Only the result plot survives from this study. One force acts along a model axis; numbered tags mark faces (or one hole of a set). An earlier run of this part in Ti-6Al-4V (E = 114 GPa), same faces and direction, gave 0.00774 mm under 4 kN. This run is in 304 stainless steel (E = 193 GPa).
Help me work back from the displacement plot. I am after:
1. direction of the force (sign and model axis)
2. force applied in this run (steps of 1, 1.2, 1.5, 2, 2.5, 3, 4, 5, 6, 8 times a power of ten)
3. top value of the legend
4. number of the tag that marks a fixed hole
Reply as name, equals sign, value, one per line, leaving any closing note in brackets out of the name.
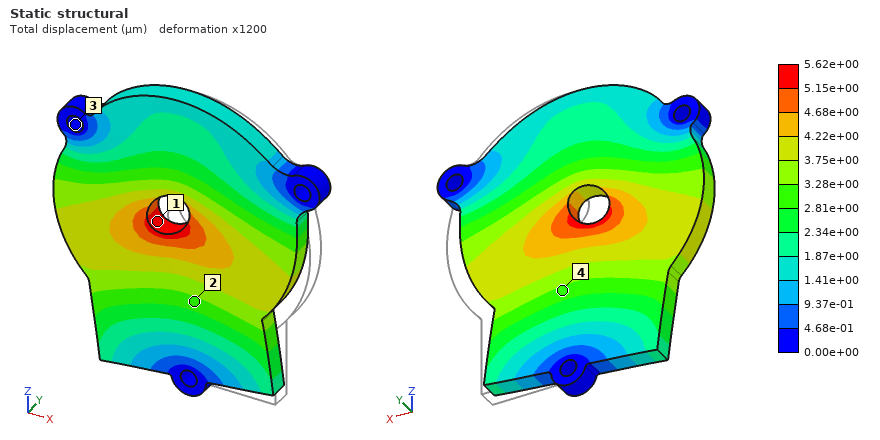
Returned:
direction of the force = -X
force applied in this run = 5 kN
top value of the legend = 5.62e+00 µm
number of the tag that marks a fixed hole = 3
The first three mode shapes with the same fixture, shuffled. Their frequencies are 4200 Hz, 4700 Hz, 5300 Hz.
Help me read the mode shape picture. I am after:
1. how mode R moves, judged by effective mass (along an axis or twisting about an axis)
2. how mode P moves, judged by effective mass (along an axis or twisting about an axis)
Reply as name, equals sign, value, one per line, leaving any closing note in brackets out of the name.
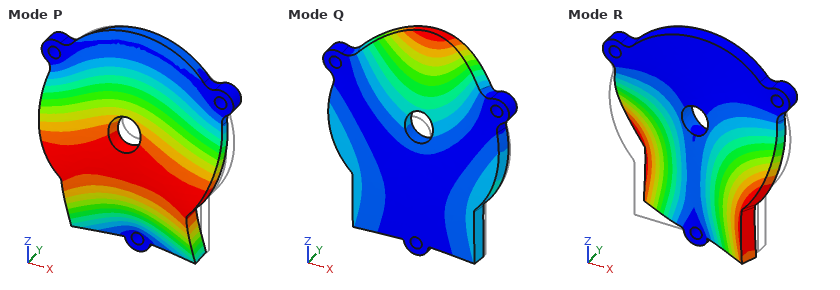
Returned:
how mode R moves, judged by effective mass = twisting about Z
how mode P moves, judged by effective mass = along Y
